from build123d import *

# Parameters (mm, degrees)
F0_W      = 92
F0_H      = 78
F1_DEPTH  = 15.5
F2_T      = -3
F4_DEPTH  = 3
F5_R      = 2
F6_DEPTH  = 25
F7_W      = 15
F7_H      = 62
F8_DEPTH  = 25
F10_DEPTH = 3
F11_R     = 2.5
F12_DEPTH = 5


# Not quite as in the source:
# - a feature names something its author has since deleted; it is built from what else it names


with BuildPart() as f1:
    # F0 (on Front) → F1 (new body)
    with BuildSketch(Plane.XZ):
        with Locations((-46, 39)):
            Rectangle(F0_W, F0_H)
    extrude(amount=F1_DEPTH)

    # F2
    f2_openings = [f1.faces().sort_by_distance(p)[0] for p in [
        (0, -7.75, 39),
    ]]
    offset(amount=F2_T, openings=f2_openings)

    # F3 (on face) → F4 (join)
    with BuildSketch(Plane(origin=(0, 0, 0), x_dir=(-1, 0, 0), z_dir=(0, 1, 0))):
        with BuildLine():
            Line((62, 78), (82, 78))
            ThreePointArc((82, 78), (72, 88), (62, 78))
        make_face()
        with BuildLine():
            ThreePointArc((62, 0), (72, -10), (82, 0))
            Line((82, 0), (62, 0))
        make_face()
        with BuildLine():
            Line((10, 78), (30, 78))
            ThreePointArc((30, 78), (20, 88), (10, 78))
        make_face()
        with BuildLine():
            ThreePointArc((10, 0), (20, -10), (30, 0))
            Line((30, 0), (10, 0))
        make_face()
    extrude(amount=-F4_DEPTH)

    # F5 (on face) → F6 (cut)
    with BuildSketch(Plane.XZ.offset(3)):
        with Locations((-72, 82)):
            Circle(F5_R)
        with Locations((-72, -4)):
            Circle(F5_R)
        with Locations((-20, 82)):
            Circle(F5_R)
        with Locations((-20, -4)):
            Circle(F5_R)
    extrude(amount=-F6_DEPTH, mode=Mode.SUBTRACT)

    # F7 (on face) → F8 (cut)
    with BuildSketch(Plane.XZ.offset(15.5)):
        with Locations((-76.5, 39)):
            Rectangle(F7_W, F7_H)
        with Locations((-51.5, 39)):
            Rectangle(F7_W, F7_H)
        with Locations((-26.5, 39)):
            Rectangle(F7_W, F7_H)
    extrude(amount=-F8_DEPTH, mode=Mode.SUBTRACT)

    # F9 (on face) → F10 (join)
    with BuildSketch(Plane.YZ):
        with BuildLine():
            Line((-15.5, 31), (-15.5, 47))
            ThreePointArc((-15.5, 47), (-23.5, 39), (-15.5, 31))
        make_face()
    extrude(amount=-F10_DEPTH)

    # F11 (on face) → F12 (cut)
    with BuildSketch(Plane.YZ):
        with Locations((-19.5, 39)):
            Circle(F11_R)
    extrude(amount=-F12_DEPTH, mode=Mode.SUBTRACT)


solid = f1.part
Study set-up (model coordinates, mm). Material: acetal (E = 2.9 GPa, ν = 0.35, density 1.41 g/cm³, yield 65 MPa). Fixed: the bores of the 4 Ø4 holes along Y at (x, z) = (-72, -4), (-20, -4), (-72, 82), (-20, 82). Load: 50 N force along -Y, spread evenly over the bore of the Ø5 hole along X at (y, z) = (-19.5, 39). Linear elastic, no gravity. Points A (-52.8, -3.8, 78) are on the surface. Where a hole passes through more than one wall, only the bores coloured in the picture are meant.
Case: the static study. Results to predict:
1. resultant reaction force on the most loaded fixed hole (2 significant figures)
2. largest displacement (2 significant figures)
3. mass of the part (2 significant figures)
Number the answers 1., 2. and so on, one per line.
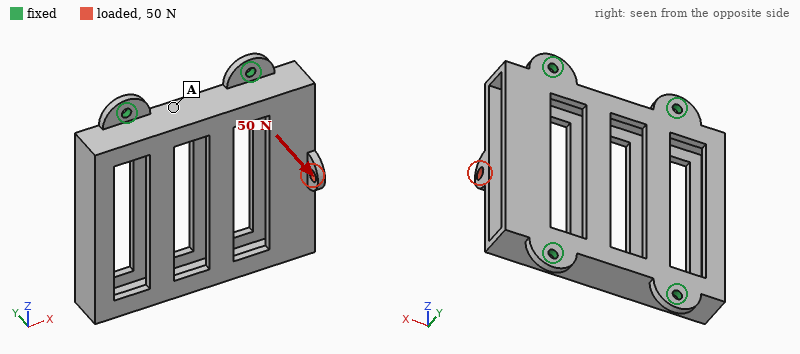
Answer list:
1. 42 N
2. 1.1 mm
3. 50 g
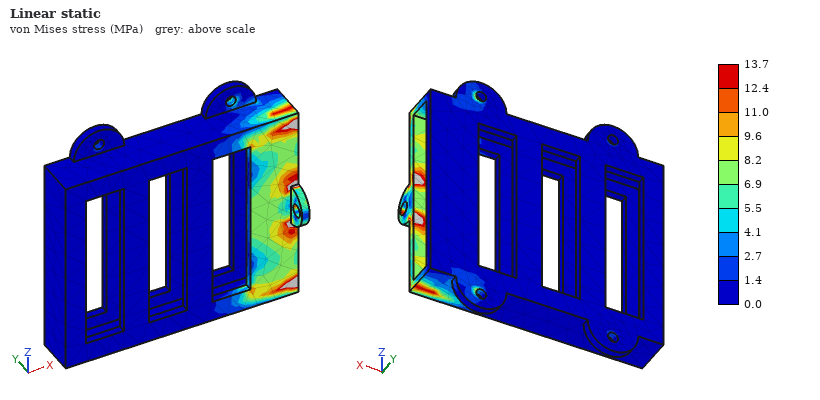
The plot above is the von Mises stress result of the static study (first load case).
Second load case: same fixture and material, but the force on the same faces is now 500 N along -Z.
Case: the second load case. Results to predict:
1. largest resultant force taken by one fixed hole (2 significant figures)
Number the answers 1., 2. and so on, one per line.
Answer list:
1. 260 N
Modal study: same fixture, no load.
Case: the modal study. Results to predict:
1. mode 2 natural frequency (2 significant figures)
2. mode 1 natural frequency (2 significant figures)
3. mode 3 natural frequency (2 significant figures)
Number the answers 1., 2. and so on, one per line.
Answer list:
1. 740 Hz
2. 720 Hz
3. 800 Hz
